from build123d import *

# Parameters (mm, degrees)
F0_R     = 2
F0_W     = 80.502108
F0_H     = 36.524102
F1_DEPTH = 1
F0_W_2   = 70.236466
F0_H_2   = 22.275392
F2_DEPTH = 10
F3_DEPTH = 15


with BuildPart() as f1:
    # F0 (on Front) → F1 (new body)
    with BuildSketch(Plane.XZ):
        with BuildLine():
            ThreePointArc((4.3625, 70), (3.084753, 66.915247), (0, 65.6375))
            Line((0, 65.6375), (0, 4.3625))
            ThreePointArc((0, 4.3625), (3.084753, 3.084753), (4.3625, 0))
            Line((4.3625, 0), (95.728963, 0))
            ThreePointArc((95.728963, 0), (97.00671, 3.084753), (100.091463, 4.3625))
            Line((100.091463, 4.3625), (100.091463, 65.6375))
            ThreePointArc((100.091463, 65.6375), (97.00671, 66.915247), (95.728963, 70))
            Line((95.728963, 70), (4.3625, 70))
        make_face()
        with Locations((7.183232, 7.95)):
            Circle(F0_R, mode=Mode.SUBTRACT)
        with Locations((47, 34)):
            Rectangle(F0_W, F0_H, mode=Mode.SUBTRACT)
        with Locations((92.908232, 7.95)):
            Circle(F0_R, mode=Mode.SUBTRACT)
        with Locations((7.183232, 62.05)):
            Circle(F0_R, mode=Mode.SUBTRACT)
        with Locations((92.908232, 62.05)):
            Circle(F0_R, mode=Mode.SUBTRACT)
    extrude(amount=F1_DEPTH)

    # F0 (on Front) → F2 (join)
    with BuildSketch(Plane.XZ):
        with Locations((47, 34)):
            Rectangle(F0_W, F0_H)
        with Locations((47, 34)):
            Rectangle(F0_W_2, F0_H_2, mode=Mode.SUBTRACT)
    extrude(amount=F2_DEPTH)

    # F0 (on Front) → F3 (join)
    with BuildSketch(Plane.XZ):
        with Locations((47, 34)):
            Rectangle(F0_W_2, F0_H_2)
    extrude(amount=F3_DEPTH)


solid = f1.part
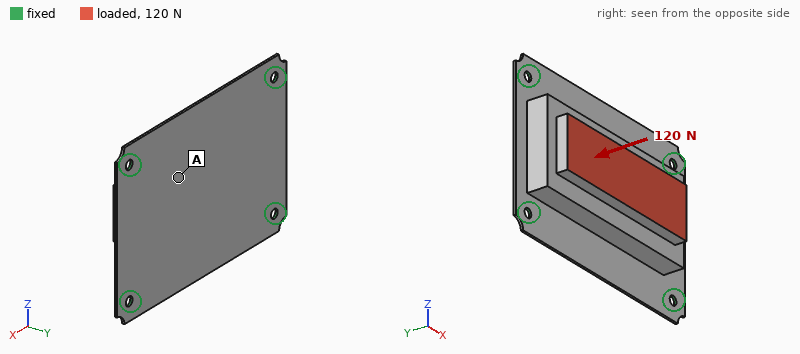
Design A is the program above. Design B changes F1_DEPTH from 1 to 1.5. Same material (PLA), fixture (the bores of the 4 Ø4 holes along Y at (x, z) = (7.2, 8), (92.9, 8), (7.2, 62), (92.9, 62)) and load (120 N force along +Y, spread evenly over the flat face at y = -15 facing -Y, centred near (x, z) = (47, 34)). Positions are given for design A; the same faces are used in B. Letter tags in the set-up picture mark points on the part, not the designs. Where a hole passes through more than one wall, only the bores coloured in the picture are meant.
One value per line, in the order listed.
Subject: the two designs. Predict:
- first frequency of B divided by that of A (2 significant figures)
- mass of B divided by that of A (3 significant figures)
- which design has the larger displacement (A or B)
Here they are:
1.5
1.05
A
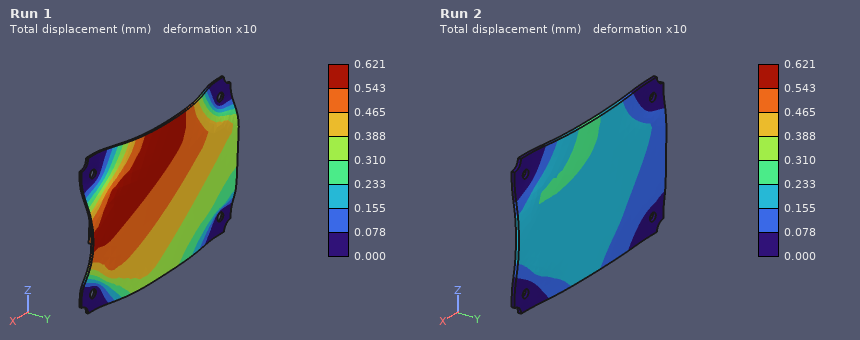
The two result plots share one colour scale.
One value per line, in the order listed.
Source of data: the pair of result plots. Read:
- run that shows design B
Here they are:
Run 2
